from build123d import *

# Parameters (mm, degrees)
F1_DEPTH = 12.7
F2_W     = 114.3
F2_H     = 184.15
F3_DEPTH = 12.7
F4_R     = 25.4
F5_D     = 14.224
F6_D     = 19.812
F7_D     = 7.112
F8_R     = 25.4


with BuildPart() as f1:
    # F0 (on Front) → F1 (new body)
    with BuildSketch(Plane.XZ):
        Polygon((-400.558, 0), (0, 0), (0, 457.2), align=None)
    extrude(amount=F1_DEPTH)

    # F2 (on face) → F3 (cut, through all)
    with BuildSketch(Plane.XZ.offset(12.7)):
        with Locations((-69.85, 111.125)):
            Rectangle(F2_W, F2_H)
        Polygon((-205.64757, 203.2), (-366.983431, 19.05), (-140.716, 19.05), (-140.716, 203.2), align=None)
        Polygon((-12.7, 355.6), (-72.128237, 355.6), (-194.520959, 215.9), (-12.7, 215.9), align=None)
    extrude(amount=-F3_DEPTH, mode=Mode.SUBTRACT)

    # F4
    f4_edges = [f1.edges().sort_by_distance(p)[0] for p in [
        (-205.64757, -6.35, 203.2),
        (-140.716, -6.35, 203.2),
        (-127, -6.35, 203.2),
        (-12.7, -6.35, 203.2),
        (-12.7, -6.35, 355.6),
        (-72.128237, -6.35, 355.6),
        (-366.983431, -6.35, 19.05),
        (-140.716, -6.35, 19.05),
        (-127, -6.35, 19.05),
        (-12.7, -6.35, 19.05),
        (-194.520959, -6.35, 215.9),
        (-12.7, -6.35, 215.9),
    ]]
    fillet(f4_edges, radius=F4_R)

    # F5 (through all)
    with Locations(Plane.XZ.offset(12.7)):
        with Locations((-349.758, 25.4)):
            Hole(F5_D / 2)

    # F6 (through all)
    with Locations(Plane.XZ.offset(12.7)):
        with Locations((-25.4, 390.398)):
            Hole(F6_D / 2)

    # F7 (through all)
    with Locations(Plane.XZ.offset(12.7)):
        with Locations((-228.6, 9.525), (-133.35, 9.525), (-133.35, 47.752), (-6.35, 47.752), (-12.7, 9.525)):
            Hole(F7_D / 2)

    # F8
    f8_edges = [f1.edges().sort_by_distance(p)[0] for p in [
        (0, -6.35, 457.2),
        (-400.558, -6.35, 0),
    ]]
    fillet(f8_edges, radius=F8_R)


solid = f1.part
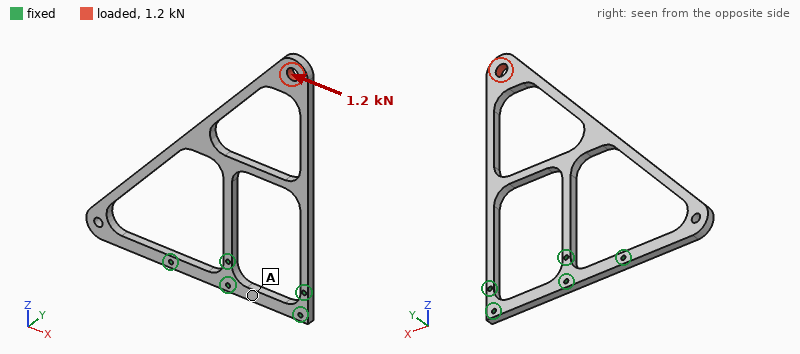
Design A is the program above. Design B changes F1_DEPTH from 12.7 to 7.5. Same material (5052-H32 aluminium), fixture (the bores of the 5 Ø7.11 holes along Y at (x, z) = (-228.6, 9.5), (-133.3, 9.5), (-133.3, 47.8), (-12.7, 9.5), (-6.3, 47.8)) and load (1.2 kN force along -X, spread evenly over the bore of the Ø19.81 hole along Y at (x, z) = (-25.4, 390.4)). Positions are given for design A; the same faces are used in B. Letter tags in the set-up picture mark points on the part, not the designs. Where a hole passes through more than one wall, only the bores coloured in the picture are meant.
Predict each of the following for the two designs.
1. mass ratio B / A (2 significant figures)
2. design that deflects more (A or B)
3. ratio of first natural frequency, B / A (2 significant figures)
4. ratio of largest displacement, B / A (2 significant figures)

0.59
B
0.60
1.7
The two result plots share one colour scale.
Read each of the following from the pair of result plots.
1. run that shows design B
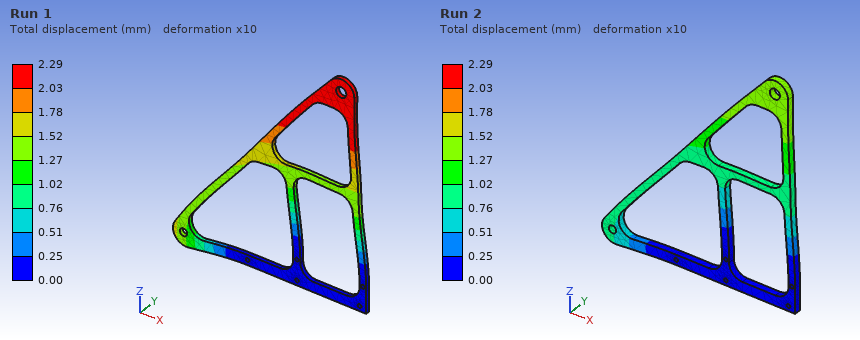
Run 1
